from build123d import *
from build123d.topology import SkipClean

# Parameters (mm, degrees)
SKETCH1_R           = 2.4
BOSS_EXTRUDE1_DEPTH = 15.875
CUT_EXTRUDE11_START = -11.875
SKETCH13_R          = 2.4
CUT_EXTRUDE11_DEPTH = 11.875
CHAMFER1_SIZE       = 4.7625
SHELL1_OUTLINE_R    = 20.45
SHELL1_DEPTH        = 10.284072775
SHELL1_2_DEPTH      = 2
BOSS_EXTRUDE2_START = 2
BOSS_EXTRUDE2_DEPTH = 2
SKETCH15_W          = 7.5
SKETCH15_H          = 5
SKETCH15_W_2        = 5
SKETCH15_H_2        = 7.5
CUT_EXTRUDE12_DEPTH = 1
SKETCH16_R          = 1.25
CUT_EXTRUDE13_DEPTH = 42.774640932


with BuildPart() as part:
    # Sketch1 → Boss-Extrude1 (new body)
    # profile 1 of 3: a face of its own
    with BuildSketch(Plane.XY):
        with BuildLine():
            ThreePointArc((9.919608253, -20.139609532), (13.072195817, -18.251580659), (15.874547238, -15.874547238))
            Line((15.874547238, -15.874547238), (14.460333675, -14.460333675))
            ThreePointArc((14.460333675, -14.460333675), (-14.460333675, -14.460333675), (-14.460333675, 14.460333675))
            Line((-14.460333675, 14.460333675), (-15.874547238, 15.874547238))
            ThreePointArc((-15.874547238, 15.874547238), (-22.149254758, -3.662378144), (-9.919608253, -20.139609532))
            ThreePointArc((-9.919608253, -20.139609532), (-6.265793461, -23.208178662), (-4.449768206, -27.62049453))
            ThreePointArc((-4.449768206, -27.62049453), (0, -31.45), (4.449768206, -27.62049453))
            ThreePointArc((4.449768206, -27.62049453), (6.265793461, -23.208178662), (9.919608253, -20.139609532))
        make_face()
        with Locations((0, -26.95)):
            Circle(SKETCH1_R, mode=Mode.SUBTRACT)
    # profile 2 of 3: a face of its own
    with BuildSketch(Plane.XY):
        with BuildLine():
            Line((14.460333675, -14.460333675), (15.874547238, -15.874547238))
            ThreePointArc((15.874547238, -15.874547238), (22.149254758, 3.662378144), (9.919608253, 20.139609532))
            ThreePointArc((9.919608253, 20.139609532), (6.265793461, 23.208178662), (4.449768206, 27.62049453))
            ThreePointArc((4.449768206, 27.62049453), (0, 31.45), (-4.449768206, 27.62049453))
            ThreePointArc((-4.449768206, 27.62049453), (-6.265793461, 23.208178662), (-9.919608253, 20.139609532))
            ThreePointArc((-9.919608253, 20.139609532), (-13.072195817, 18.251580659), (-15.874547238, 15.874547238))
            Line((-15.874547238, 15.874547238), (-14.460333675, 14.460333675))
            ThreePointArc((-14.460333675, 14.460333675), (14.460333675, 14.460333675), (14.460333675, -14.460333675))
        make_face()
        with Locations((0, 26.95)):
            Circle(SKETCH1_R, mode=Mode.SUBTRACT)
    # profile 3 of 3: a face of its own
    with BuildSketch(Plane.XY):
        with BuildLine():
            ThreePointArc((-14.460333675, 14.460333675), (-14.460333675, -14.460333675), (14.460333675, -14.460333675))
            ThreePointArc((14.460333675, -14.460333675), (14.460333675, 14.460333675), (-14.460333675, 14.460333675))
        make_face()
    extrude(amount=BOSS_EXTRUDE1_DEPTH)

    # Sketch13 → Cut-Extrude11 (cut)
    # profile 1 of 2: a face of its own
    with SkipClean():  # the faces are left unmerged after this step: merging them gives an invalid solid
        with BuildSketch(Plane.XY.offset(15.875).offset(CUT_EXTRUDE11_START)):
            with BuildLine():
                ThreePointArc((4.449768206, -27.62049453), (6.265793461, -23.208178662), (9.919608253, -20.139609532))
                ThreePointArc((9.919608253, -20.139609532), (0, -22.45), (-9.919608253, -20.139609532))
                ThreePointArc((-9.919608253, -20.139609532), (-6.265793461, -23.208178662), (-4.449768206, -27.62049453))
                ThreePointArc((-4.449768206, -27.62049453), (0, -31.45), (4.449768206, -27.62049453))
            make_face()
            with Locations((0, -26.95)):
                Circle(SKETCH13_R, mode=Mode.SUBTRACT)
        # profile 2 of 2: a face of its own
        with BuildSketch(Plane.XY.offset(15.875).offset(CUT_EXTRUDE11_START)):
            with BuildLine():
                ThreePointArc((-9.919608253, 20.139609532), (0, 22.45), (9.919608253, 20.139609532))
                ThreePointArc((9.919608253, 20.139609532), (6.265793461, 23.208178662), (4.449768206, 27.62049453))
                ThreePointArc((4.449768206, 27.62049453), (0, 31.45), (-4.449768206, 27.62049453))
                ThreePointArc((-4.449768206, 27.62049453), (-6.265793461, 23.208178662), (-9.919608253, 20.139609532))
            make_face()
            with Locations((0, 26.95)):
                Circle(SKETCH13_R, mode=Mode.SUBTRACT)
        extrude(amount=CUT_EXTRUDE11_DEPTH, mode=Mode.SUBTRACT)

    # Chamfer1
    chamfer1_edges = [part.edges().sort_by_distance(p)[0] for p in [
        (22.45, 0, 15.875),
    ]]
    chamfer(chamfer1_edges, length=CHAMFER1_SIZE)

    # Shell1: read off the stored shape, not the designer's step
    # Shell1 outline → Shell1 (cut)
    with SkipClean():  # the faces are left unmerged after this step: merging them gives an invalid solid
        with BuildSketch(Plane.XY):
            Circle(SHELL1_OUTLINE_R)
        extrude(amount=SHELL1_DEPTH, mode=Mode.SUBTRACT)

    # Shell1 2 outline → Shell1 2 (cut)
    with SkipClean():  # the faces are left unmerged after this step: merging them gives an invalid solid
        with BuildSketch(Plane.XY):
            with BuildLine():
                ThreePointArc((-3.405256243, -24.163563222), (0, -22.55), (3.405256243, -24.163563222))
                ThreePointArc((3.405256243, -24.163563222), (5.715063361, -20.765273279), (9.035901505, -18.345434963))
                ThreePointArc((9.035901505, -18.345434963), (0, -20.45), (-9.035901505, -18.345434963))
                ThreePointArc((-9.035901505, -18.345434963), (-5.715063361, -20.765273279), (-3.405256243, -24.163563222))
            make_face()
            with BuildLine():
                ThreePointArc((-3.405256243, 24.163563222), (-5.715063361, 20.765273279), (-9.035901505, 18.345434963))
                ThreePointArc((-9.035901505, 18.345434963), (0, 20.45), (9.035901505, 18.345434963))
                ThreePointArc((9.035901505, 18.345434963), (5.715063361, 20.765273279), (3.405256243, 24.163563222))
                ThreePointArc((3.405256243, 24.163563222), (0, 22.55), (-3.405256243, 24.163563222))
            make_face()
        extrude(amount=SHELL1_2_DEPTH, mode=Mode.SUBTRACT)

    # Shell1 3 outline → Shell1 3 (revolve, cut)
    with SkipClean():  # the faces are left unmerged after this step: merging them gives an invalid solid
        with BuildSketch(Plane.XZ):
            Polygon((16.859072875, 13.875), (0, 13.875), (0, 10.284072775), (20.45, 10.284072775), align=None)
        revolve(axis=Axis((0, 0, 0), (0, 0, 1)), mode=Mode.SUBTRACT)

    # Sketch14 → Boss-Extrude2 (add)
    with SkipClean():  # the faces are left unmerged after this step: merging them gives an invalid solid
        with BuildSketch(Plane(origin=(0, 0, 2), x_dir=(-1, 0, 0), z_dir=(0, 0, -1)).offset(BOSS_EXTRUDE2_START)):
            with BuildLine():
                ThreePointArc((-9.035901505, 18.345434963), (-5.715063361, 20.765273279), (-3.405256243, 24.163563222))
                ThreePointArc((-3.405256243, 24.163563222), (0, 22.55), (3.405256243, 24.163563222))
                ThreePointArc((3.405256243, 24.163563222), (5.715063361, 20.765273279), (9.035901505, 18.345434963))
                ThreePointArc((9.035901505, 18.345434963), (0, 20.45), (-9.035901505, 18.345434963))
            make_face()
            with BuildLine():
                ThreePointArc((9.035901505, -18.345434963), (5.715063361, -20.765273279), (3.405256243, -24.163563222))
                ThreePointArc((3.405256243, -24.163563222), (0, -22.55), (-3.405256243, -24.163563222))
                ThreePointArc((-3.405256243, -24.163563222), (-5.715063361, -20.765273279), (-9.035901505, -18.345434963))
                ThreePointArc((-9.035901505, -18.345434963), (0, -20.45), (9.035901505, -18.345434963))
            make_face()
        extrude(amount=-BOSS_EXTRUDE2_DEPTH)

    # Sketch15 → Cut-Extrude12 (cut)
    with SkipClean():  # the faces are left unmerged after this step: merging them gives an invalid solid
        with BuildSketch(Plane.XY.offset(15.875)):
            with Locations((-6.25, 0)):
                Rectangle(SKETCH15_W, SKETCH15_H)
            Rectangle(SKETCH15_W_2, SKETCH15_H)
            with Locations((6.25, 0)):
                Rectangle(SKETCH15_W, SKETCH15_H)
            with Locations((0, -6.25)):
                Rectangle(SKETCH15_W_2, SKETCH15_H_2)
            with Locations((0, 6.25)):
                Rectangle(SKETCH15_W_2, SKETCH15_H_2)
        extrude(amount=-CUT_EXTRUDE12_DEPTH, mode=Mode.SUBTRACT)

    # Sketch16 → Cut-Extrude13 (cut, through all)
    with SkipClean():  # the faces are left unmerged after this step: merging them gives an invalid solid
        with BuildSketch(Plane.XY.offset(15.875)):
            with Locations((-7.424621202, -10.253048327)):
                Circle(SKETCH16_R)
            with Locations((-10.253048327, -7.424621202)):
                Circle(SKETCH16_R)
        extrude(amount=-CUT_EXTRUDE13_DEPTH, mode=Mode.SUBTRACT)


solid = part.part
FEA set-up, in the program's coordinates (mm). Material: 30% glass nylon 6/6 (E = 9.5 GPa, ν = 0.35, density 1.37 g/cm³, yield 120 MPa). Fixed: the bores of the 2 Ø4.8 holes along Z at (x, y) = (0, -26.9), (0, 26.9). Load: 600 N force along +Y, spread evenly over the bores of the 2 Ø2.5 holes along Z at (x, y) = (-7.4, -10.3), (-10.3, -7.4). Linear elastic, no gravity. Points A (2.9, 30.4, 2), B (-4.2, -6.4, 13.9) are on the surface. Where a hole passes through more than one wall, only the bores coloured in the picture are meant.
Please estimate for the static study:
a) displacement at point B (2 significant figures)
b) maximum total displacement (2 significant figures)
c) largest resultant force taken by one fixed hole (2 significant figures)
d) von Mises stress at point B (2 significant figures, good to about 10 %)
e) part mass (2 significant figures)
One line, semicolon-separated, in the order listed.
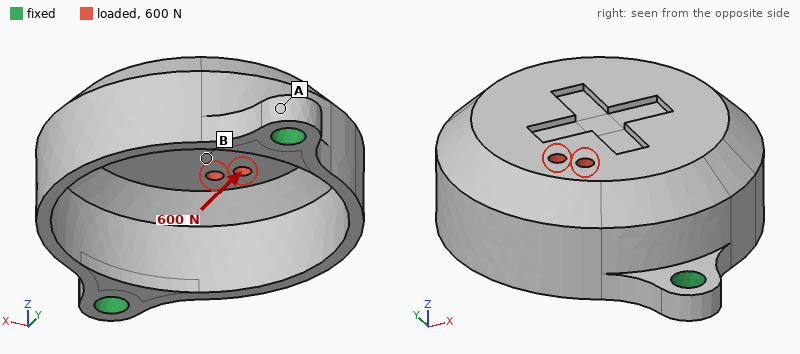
0.14 mm; 0.26 mm; 350 N; 14 MPa; 9.0 g
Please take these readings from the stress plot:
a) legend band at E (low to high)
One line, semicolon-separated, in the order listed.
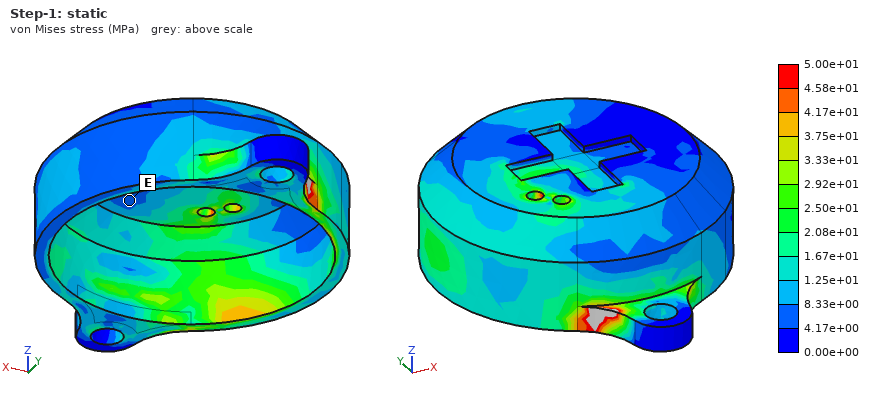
4.17e+00 to 8.33e+00 MPa
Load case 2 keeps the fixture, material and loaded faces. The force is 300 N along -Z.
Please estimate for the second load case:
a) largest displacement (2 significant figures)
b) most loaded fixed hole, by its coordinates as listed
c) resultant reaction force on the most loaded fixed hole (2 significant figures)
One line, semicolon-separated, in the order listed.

0.32 mm; (0, -26.9); 230 N
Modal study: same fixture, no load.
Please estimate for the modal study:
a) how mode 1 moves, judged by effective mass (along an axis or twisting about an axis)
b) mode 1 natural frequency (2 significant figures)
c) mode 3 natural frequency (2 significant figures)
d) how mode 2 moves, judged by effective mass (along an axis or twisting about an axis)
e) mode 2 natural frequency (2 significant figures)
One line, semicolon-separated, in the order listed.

along X; 1900 Hz; 4200 Hz; along Y; 3700 Hz
